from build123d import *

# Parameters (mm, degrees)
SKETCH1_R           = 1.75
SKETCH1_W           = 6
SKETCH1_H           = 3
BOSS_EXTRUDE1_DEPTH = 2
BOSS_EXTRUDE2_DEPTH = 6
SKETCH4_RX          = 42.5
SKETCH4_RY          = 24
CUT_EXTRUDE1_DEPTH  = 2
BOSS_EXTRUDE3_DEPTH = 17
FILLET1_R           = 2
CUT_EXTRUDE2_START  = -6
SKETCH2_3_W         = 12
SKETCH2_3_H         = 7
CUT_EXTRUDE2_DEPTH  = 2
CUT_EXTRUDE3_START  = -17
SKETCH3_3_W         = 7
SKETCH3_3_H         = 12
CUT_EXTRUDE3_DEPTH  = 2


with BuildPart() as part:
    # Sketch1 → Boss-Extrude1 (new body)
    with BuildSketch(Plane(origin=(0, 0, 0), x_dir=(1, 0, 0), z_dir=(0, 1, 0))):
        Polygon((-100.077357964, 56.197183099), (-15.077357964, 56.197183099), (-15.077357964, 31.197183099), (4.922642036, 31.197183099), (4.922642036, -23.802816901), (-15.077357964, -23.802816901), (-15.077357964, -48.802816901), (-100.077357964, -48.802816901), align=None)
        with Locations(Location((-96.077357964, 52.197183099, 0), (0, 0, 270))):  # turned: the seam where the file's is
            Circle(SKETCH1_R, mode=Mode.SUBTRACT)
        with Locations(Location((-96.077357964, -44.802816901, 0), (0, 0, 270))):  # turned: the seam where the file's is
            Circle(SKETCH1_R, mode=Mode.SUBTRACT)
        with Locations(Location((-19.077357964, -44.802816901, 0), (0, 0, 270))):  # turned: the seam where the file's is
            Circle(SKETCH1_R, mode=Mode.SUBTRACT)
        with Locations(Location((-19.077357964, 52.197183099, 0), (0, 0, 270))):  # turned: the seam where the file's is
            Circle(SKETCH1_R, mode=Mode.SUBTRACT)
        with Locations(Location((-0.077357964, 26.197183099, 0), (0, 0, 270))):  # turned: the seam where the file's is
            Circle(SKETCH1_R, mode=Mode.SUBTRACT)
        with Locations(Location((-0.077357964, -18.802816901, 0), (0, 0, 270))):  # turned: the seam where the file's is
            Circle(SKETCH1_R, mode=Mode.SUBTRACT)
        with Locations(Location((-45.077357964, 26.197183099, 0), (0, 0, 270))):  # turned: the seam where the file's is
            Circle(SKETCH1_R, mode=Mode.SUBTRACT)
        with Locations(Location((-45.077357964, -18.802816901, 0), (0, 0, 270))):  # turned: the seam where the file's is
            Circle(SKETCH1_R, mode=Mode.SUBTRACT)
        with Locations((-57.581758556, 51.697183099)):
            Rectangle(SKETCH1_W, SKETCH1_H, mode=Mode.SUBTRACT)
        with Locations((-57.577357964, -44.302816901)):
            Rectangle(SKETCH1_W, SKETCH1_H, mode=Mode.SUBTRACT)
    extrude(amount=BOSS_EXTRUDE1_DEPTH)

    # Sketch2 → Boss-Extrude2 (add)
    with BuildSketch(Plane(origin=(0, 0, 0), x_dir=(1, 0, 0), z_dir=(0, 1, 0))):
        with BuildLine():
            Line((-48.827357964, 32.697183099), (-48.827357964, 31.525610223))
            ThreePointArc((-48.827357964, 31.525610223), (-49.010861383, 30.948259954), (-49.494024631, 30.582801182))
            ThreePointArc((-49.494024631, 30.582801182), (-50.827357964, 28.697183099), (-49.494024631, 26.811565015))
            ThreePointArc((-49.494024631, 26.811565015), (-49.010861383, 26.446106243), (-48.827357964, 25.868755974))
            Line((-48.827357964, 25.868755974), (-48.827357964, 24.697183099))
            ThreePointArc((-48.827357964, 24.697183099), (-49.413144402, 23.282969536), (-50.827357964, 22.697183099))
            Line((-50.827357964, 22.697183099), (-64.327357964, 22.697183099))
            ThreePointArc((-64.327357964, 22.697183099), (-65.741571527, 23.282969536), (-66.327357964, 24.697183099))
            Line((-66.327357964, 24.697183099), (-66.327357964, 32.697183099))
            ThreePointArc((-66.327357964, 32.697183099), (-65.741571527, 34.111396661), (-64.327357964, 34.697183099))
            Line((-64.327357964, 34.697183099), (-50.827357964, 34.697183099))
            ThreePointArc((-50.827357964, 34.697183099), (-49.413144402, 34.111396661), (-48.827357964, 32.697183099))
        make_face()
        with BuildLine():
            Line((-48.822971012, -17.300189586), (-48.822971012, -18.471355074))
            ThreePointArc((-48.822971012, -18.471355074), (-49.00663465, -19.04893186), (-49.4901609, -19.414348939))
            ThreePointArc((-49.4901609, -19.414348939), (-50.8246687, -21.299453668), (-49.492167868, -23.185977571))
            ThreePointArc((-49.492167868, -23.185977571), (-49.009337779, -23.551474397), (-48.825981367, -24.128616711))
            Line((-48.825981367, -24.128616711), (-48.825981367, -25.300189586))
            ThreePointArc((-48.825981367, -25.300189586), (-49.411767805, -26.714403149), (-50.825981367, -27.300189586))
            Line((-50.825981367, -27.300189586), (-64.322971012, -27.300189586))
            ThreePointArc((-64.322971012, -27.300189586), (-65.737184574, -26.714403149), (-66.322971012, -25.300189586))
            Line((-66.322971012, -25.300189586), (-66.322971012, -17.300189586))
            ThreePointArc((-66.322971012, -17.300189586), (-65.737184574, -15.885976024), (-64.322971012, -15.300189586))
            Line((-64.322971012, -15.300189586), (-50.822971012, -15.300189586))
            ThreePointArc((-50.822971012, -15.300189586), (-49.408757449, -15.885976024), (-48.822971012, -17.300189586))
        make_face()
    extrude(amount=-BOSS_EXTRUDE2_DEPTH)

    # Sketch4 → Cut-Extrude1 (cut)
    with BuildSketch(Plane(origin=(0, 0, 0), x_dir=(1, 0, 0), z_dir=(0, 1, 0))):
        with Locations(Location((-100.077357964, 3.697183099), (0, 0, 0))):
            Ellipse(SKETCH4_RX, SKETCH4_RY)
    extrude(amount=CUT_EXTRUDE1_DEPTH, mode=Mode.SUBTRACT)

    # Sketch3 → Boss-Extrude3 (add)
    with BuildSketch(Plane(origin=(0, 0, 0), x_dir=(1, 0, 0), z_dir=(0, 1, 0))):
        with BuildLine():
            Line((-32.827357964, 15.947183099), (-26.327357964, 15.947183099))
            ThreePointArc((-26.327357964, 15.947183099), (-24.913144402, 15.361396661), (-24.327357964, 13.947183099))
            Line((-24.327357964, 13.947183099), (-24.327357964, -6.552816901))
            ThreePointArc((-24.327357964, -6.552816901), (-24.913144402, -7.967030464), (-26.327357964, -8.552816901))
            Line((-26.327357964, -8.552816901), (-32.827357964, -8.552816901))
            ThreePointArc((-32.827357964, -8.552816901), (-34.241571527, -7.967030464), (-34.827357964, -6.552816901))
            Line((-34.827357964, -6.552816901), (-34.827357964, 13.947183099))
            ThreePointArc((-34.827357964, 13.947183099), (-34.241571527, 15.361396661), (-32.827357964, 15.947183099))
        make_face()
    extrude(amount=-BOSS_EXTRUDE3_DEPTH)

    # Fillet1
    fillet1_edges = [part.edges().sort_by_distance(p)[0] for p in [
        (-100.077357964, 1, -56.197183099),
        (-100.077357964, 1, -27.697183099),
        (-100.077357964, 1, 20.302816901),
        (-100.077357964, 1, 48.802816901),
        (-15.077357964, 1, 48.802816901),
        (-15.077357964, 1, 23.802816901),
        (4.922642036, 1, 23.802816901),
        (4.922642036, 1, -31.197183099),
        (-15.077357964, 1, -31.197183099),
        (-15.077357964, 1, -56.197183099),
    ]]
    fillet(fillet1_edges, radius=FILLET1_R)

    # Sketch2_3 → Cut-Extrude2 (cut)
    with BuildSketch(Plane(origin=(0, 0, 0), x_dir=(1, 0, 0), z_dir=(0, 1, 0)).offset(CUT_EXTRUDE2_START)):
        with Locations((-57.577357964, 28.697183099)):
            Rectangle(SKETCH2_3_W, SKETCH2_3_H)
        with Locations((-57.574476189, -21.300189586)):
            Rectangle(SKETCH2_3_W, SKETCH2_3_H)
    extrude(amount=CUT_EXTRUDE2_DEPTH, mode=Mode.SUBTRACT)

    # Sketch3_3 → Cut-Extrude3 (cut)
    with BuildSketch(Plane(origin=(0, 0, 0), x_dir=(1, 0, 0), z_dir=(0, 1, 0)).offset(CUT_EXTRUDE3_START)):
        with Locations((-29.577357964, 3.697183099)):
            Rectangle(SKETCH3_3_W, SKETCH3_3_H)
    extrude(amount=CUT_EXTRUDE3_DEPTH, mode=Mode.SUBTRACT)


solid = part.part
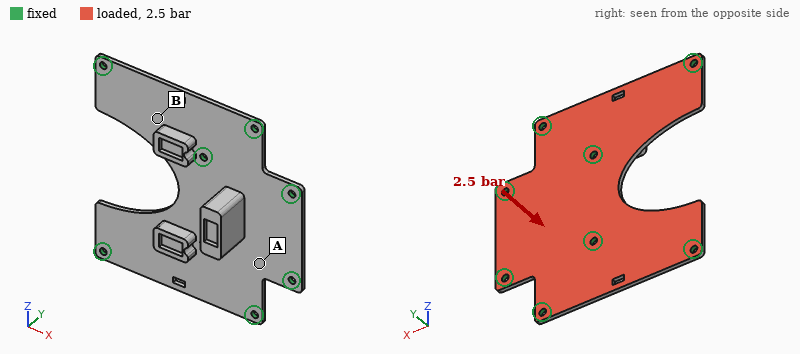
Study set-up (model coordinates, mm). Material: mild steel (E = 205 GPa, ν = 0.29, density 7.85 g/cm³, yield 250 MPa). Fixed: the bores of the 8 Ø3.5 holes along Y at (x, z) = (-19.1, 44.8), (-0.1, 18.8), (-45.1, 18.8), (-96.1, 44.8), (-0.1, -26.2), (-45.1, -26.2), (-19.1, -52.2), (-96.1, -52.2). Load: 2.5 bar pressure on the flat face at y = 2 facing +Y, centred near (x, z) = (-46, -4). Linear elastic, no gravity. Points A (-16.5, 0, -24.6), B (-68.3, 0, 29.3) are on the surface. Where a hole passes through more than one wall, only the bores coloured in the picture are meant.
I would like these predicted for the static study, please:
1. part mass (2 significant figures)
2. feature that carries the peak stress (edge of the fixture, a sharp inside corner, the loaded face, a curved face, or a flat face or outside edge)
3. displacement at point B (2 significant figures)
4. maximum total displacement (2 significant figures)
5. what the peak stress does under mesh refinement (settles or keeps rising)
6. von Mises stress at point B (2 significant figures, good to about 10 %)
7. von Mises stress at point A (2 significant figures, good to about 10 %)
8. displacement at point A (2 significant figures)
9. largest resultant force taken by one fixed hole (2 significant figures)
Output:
180 g
edge of the fixture
60 µm
80 µm
keeps rising
56 MPa
25 MPa
18 µm
530 N
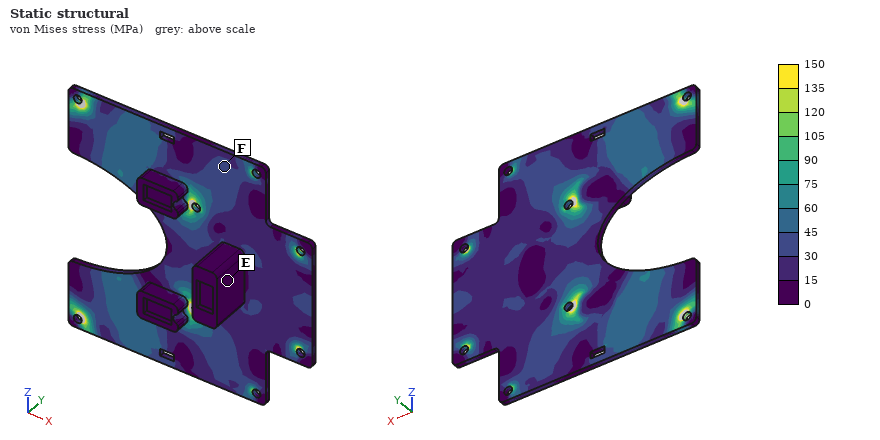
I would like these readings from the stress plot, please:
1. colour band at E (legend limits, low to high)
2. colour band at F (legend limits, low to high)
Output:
0 to 15 MPa
30 to 45 MPa
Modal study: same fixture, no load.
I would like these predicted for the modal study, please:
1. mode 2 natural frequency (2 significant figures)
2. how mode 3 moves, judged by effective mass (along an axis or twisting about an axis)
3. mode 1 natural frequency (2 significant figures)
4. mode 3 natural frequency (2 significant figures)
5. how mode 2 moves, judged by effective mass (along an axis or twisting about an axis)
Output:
2600 Hz
along Y
2500 Hz
2700 Hz
twisting about X
